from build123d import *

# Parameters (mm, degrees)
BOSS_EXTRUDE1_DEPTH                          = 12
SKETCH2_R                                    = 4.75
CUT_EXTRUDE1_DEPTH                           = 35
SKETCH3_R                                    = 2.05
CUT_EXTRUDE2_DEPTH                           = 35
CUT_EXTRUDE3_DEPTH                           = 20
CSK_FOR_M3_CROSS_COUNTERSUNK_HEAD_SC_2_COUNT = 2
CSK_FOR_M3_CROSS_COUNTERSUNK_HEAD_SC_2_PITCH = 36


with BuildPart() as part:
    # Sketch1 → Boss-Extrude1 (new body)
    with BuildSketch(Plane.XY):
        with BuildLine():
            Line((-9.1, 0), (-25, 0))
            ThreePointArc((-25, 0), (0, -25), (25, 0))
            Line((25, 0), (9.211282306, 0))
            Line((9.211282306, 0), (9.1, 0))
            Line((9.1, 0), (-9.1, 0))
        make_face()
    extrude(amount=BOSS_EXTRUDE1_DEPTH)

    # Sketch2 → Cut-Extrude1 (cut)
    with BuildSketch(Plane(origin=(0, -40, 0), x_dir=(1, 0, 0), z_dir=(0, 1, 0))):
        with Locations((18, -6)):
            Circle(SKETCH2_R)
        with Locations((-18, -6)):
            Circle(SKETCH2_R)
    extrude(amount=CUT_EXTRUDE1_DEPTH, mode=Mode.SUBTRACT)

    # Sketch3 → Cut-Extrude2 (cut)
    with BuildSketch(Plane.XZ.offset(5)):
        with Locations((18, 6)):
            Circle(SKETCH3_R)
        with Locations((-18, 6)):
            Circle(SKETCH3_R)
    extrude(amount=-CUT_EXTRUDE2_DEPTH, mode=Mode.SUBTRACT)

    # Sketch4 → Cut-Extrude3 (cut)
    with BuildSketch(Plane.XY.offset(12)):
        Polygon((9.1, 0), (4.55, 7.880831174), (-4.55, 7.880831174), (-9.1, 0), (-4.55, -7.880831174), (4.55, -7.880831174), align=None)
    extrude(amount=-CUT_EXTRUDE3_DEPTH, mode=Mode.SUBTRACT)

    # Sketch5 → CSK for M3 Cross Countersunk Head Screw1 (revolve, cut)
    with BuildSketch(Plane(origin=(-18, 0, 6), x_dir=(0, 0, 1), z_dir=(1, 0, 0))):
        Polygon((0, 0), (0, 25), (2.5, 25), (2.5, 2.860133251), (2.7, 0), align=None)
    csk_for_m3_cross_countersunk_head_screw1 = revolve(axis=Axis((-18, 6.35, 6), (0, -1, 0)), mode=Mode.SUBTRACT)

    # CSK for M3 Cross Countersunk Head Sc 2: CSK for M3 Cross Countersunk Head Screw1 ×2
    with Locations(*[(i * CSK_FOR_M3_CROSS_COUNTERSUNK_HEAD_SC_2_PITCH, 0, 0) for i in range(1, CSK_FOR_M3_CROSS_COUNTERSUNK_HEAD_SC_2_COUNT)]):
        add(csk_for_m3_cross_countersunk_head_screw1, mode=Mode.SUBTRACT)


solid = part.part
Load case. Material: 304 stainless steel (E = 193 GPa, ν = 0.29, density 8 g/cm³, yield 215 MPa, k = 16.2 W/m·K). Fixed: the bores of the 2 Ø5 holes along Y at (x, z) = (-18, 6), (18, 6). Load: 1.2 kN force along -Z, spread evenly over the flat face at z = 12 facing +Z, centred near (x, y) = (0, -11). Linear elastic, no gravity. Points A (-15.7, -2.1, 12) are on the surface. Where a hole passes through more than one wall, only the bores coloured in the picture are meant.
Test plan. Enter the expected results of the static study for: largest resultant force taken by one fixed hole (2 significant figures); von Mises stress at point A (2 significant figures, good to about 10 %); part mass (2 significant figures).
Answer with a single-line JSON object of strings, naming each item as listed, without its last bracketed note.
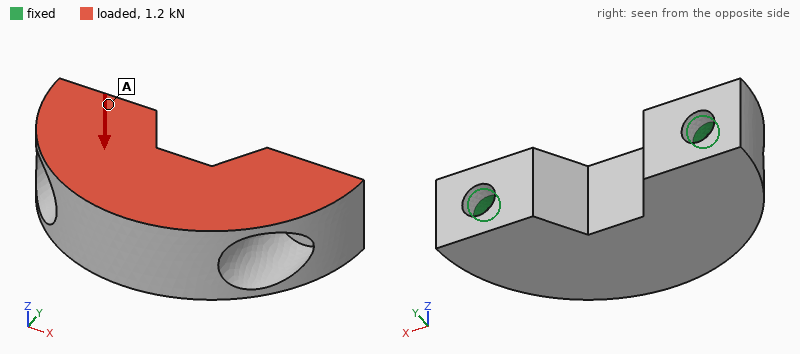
{"largest resultant force taken by one fixed hole": "600 N", "von Mises stress at point A": "24 MPa", "part mass": "69 g"}
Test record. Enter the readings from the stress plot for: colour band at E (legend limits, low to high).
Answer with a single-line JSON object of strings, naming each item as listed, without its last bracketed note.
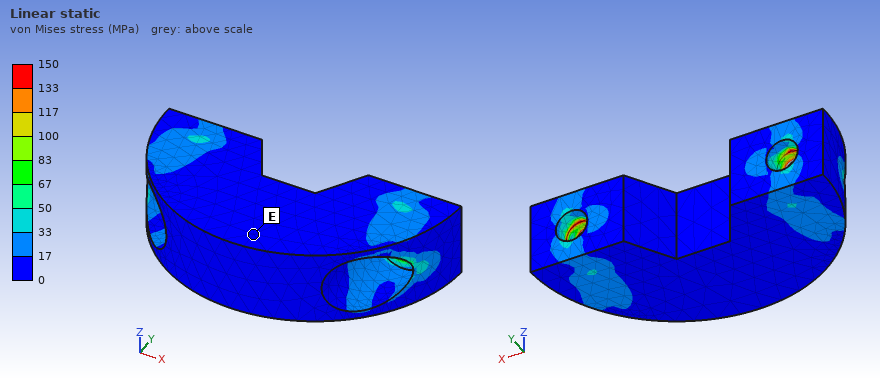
{"colour band at E": "0 to 17 MPa"}
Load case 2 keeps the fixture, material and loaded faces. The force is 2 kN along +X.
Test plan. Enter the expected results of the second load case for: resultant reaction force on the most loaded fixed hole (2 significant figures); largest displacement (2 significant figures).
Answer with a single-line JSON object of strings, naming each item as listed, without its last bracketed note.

{"resultant reaction force on the most loaded fixed hole": "1.1 kN", "largest displacement": "3.6 µm"}
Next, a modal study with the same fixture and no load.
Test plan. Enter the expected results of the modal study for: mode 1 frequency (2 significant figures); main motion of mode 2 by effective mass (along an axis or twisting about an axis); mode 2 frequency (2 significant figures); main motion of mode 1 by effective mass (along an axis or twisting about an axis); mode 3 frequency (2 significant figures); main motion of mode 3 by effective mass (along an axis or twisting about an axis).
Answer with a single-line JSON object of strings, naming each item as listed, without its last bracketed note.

{"mode 1 frequency": "5900 Hz", "main motion of mode 2 by effective mass": "along Y", "mode 2 frequency": "20 kHz", "main motion of mode 1 by effective mass": "along Z", "mode 3 frequency": "21 kHz", "main motion of mode 3 by effective mass": "twisting about Y"}
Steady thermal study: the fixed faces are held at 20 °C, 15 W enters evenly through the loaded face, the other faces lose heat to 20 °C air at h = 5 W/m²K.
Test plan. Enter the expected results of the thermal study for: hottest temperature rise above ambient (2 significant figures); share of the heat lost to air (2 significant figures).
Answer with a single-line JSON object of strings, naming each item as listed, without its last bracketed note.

{"hottest temperature rise above ambient": "57 K", "share of the heat lost to air": "3.4 %"}
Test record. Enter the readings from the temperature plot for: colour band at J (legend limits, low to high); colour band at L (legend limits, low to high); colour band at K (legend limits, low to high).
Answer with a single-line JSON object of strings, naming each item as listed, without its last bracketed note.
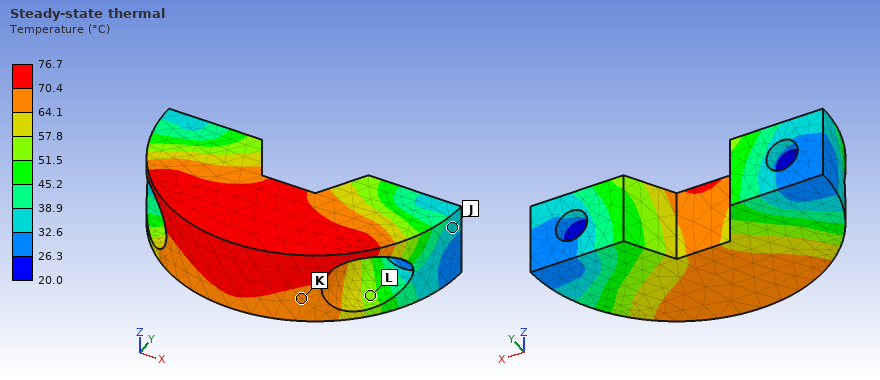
{"colour band at J": "32.6 to 38.9 °C", "colour band at L": "51.5 to 57.8 °C", "colour band at K": "64.1 to 70.4 °C"}
